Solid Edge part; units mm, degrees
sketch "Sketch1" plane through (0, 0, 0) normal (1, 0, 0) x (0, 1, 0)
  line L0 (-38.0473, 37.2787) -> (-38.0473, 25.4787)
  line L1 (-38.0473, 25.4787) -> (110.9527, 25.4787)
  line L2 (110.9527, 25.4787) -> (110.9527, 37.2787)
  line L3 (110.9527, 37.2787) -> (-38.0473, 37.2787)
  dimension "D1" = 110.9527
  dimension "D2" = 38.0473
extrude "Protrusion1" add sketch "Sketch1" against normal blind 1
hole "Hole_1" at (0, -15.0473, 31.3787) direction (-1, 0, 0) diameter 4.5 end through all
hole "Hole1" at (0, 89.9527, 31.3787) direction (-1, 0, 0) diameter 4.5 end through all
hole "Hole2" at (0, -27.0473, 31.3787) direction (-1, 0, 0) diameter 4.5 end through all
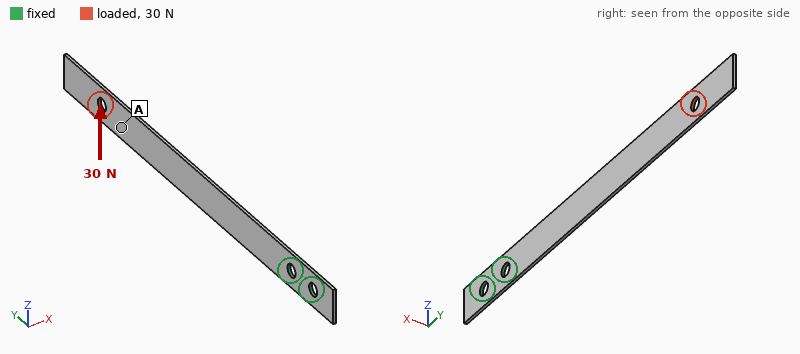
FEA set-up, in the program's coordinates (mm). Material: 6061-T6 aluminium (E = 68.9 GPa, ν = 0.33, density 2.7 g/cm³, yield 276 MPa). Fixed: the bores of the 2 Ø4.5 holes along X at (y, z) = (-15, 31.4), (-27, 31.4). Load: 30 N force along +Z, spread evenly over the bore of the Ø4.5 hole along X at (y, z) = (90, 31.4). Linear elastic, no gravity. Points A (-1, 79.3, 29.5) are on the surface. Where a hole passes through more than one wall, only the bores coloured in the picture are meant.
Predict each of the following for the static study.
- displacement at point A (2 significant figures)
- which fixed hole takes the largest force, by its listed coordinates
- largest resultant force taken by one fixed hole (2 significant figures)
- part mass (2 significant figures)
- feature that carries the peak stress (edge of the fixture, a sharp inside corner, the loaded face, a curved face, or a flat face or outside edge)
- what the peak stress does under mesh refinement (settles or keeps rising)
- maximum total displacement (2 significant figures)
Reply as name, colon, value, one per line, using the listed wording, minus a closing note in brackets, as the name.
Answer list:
displacement at point A: 1.1 mm
which fixed hole takes the largest force, by its listed coordinates: (-15, 31.4)
largest resultant force taken by one fixed hole: 130 N
part mass: 4.6 g
feature that carries the peak stress: edge of the fixture
what the peak stress does under mesh refinement: keeps rising
maximum total displacement: 1.7 mm
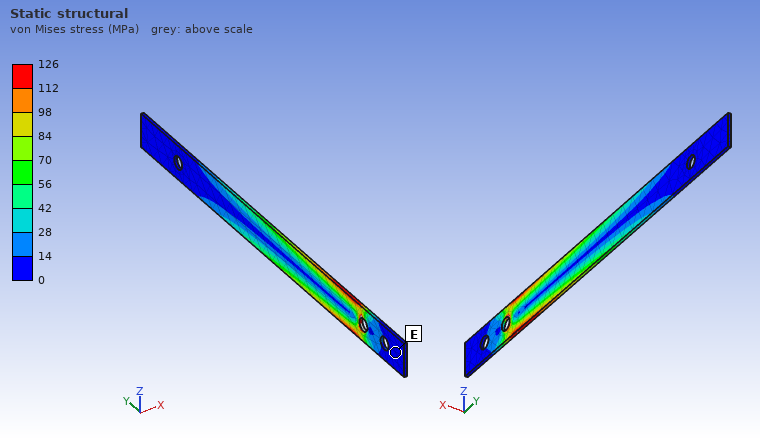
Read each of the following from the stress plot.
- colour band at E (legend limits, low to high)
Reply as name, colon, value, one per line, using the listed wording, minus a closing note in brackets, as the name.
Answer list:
colour band at E: 0 to 14 MPa
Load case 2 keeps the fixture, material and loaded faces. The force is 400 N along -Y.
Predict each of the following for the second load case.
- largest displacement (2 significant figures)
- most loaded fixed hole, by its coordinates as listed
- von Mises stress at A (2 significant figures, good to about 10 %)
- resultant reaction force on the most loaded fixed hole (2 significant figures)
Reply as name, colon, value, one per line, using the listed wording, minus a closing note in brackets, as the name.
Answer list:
largest displacement: 54 µm
most loaded fixed hole, by its coordinates as listed: (-15, 31.4)
von Mises stress at A: 34 MPa
resultant reaction force on the most loaded fixed hole: 370 N
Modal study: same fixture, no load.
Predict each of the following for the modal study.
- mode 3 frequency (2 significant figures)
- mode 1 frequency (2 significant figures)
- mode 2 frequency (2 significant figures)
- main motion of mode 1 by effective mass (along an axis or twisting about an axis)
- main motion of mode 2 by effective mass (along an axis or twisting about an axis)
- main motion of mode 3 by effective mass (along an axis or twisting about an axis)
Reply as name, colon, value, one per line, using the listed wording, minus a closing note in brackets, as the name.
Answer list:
mode 3 frequency: 590 Hz
mode 1 frequency: 54 Hz
mode 2 frequency: 330 Hz
main motion of mode 1 by effective mass: along X
main motion of mode 2 by effective mass: along X
main motion of mode 3 by effective mass: along Z
